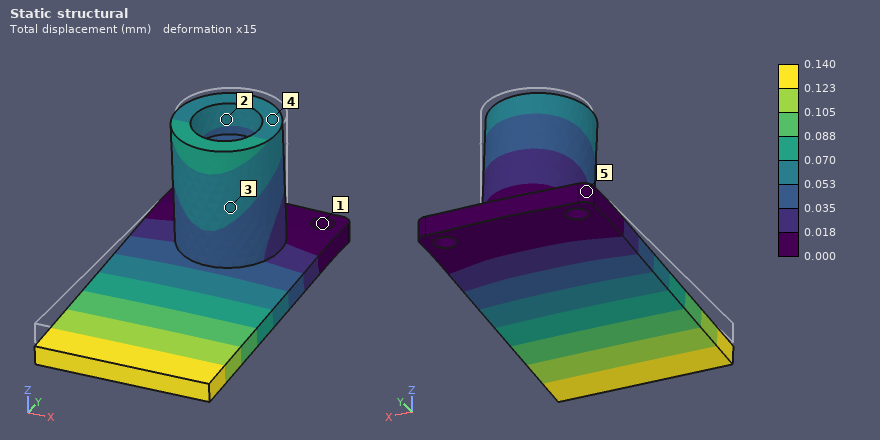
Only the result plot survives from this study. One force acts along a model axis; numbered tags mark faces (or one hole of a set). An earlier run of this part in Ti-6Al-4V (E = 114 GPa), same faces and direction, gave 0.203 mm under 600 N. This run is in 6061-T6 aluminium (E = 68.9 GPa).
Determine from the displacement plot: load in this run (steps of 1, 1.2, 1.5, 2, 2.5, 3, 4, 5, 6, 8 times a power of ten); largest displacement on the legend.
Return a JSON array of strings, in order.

["250 N", "0.140 mm"]
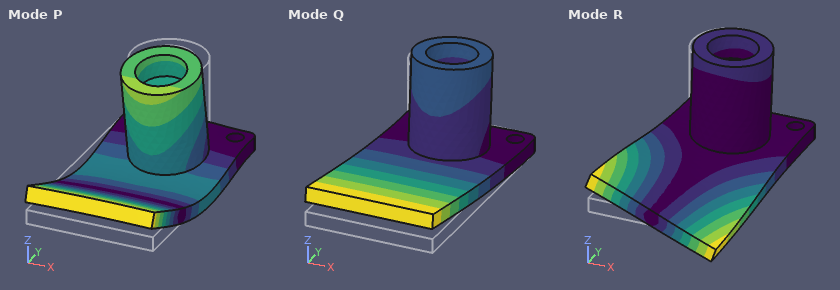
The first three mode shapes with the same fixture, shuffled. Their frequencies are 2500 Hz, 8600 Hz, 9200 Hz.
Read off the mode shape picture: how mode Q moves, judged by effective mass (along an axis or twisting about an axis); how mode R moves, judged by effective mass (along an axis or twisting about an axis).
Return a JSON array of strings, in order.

["along Z", "twisting about Y"]
